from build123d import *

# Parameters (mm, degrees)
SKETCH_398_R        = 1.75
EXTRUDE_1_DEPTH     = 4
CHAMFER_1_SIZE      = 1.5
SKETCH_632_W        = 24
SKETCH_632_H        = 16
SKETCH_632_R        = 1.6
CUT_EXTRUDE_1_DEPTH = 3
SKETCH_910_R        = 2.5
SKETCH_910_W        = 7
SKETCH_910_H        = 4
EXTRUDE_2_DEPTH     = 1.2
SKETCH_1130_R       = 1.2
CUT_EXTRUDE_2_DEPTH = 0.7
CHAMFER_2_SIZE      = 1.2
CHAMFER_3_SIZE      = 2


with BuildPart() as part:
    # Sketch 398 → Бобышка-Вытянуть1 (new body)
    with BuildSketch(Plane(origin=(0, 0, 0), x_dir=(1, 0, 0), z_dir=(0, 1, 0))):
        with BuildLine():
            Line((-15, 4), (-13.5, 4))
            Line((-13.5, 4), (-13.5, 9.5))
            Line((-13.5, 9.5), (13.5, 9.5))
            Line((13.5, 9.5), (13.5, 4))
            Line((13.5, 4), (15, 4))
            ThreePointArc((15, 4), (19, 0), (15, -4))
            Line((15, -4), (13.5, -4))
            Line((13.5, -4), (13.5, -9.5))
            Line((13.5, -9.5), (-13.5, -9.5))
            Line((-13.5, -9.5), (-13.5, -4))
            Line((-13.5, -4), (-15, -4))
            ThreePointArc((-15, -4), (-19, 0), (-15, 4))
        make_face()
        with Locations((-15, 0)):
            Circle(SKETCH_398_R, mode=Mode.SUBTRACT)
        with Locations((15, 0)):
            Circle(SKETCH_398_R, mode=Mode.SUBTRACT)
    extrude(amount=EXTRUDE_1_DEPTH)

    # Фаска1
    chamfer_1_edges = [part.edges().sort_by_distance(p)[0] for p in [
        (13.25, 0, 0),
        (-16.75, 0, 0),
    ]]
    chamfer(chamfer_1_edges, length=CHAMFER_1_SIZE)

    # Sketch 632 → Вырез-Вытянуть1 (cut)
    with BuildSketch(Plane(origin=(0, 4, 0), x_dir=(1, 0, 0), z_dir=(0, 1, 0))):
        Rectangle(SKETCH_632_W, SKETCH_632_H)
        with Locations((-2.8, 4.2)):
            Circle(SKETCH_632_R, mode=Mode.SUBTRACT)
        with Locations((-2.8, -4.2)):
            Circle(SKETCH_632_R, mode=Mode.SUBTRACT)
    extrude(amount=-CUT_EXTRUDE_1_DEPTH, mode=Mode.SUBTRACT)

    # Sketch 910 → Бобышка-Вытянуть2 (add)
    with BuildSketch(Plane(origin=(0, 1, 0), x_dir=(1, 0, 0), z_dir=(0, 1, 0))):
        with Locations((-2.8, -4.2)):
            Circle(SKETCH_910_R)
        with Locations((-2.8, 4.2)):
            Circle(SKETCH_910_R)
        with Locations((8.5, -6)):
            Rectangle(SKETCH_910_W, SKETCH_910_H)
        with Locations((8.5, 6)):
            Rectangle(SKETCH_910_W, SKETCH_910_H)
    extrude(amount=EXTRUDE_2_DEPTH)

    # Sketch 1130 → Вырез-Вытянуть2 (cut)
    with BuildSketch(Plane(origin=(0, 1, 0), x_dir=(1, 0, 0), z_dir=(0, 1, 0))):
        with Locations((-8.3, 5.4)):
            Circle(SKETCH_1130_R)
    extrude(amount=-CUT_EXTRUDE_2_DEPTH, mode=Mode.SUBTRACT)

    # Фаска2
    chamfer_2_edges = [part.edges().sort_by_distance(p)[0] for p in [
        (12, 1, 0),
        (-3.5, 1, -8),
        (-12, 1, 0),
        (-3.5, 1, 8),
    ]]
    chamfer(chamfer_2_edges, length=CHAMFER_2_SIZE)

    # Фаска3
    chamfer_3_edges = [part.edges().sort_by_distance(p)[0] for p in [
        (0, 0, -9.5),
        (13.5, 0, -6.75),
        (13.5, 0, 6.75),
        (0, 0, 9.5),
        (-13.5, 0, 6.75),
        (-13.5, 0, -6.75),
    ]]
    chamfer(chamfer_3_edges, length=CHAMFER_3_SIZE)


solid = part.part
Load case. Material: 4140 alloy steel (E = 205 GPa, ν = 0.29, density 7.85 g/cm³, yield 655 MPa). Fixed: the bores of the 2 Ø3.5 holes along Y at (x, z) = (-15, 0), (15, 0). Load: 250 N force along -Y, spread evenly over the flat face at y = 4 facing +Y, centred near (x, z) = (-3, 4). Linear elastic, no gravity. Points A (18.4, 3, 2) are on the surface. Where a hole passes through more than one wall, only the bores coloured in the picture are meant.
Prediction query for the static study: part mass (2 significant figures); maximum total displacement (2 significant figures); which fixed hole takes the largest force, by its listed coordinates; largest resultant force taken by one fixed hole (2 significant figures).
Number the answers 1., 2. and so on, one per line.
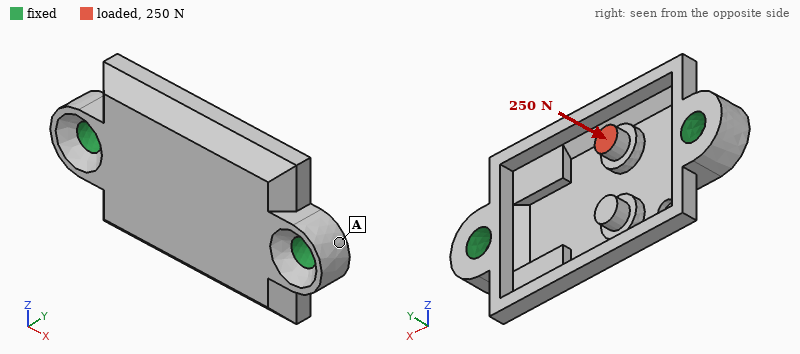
1. 8.9 g
2. 23 µm
3. (-15, 0)
4. 180 N
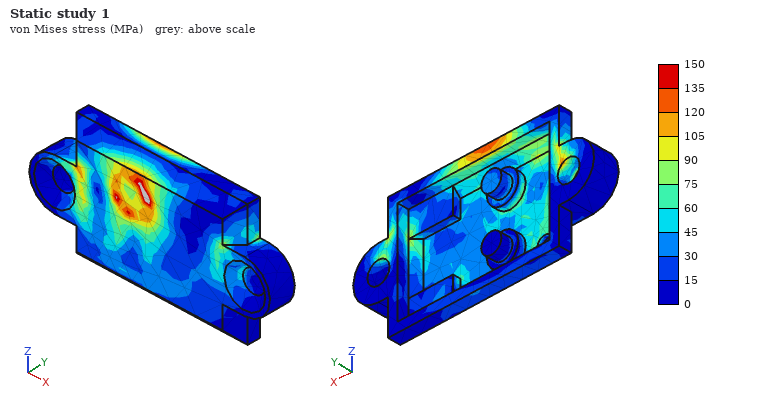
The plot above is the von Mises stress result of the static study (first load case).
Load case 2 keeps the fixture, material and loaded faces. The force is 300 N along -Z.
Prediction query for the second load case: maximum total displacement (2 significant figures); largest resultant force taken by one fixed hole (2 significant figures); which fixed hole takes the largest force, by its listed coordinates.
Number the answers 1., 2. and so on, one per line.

1. 25 µm
2. 190 N
3. (-15, 0)
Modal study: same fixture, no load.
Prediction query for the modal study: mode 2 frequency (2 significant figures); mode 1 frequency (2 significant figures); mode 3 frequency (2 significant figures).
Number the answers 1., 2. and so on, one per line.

1. 12 kHz
2. 12 kHz
3. 20 kHz
